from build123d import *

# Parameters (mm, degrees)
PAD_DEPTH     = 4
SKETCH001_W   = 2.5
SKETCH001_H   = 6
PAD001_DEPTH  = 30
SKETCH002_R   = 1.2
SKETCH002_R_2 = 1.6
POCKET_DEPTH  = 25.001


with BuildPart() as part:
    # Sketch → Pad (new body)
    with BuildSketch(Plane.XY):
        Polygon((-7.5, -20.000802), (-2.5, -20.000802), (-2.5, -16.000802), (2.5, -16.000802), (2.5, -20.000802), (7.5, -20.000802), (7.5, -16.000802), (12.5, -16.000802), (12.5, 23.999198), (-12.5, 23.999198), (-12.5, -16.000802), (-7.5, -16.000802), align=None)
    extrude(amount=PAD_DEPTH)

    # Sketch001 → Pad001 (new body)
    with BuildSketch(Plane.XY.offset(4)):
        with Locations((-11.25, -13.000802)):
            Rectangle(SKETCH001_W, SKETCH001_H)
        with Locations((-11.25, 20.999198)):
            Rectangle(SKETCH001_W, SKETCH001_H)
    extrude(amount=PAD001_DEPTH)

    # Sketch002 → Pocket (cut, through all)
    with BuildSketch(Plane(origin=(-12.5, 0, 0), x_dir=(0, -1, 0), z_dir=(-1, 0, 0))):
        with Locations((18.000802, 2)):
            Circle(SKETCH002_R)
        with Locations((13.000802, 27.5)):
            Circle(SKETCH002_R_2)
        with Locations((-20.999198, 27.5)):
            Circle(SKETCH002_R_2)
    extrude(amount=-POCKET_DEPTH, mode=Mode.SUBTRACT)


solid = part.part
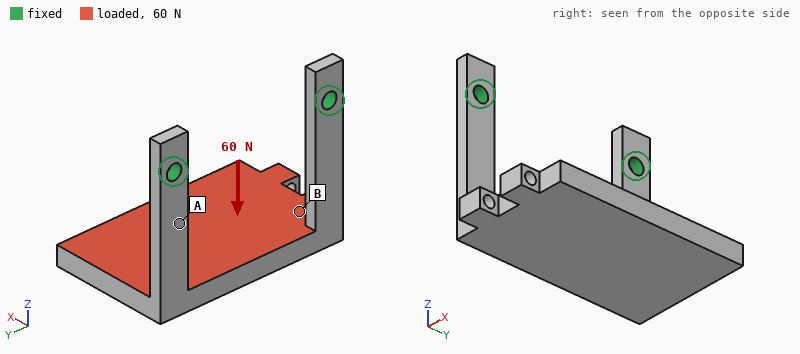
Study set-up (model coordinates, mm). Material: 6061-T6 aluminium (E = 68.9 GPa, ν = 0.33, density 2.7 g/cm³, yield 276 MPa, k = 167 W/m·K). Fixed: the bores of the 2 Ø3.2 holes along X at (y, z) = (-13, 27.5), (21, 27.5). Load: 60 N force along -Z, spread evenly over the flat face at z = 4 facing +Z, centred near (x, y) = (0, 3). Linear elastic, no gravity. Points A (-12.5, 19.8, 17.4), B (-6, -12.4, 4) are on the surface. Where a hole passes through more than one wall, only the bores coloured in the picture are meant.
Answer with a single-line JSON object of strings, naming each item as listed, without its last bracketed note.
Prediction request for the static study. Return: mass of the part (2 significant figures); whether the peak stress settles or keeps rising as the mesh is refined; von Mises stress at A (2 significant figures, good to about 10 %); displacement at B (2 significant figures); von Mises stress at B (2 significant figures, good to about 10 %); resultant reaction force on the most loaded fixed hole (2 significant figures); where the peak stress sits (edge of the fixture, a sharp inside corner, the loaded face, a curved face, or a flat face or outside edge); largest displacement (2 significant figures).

{"mass of the part": "13 g", "whether the peak stress settles or keeps rising as the mesh is refined": "keeps rising", "von Mises stress at A": "53 MPa", "displacement at B": "0.18 mm", "von Mises stress at B": "6.7 MPa", "resultant reaction force on the most loaded fixed hole": "32 N", "where the peak stress sits": "edge of the fixture", "largest displacement": "0.43 mm"}
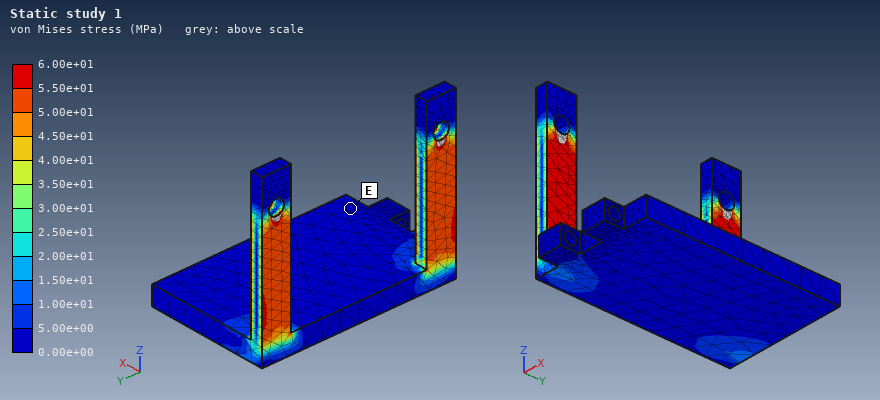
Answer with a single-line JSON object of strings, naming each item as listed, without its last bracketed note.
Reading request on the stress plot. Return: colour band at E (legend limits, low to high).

{"colour band at E": "0.00e+00 to 5.00e+00 MPa"}
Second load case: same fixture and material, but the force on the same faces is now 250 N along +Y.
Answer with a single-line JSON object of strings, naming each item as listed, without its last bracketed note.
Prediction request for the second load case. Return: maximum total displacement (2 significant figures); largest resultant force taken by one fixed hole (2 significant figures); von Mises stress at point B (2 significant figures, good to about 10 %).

{"maximum total displacement": "0.38 mm", "largest resultant force taken by one fixed hole": "160 N", "von Mises stress at point B": "42 MPa"}
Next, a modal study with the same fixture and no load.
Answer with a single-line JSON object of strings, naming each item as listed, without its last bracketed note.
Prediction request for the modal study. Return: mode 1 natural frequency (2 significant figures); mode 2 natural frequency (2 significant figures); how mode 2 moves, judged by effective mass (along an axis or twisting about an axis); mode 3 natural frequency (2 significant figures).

{"mode 1 natural frequency": "530 Hz", "mode 2 natural frequency": "1300 Hz", "how mode 2 moves, judged by effective mass": "along Y", "mode 3 natural frequency": "2000 Hz"}
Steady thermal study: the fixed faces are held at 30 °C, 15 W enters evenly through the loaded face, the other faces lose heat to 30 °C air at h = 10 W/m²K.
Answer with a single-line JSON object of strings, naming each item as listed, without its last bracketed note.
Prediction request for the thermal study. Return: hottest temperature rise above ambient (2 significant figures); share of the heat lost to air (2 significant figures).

{"hottest temperature rise above ambient": "74 K", "share of the heat lost to air": "9.5 %"}
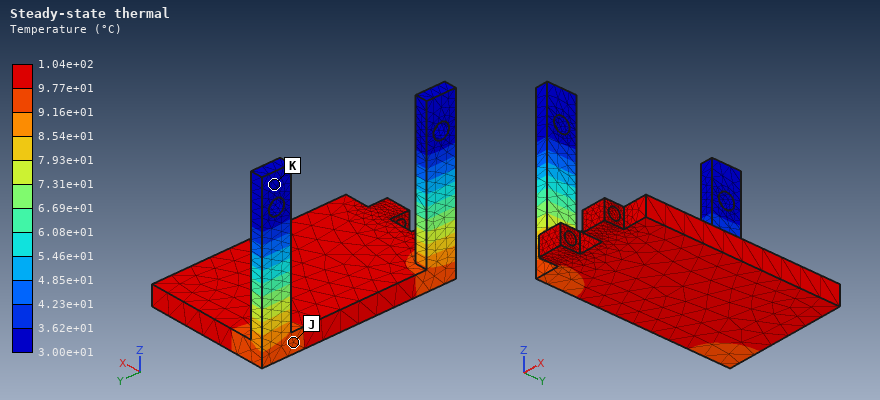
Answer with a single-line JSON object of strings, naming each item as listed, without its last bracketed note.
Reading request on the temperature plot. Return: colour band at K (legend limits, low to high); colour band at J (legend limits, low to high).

{"colour band at K": "3.00e+01 to 3.62e+01 °C", "colour band at J": "9.16e+01 to 9.77e+01 °C"}
